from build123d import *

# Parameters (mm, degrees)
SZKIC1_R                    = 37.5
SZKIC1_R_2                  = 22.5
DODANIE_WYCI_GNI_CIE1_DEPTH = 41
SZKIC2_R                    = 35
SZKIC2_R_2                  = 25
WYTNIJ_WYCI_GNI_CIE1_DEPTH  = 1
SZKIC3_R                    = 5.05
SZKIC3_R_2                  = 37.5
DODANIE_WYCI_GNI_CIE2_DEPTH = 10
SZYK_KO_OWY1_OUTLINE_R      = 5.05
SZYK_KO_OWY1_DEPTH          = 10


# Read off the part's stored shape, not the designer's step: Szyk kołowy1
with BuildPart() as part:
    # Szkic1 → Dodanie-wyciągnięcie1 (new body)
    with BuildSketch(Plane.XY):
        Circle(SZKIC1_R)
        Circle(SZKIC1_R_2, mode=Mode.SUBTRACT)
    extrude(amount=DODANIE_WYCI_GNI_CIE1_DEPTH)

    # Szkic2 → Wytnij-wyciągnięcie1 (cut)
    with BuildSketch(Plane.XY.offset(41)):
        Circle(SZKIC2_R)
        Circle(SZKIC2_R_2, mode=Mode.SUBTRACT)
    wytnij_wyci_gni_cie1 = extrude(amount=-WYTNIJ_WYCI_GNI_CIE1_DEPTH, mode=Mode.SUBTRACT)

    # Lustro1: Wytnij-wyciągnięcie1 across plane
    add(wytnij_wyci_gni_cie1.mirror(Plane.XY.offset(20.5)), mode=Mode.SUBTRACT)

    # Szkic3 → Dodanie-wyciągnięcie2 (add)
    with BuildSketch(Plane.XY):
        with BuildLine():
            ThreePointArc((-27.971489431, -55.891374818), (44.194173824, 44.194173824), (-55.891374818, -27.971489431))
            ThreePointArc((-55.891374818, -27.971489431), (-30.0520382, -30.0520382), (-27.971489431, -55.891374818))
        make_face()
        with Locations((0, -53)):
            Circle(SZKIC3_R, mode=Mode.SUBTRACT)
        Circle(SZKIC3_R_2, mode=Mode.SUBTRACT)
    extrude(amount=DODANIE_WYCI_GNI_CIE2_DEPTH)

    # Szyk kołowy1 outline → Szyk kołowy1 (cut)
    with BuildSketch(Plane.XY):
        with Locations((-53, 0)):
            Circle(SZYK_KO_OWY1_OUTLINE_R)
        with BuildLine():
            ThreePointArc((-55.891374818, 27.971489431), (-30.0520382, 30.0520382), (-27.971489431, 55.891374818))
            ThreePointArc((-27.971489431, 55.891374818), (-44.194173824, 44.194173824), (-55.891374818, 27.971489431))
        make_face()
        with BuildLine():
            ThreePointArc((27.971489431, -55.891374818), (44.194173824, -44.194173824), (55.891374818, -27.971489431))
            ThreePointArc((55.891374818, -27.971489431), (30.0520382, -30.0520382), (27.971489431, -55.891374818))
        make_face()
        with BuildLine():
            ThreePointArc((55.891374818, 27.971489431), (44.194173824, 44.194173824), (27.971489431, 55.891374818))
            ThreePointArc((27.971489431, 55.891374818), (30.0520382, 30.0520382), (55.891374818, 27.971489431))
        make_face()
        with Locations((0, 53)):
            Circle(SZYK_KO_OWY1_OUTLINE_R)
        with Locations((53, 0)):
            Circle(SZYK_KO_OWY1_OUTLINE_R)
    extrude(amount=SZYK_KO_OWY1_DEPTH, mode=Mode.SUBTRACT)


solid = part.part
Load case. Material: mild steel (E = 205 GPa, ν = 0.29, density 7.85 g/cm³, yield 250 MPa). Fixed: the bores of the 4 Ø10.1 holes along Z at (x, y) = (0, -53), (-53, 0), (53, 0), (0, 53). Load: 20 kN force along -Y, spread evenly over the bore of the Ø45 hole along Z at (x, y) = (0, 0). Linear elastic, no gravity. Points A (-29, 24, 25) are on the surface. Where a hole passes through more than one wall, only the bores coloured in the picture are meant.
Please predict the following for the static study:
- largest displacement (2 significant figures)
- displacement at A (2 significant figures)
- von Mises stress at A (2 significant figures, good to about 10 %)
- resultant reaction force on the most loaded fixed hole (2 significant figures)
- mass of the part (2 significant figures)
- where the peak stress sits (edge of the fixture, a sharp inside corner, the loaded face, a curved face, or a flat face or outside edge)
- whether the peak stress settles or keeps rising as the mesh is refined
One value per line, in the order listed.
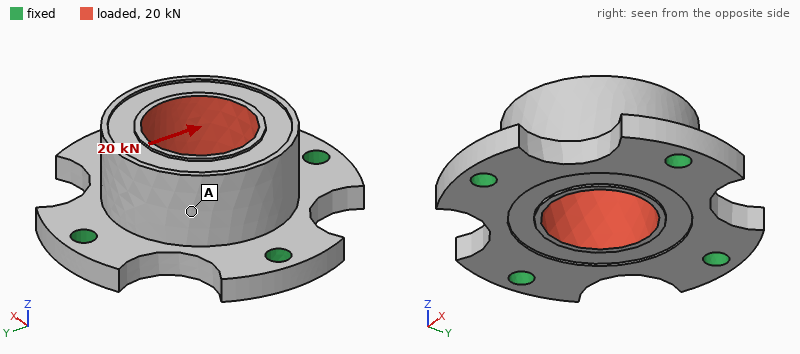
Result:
10 µm
7.0 µm
5.4 MPa
7.8 kN
1.3 kg
edge of the fixture
keeps rising
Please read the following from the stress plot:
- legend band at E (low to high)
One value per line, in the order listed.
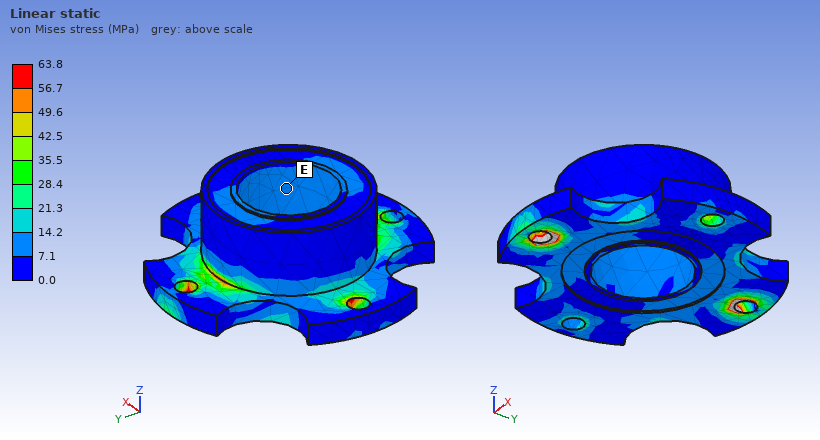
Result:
7.1 to 14.2 MPa
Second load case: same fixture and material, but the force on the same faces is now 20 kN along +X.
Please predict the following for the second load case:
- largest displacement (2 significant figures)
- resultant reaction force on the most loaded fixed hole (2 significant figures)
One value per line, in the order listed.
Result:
11 µm
7.8 kN
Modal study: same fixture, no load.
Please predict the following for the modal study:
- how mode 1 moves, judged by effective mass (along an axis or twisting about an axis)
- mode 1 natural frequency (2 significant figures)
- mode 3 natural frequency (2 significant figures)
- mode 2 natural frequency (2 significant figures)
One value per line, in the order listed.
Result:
along Z
7100 Hz
7500 Hz
7500 Hz
